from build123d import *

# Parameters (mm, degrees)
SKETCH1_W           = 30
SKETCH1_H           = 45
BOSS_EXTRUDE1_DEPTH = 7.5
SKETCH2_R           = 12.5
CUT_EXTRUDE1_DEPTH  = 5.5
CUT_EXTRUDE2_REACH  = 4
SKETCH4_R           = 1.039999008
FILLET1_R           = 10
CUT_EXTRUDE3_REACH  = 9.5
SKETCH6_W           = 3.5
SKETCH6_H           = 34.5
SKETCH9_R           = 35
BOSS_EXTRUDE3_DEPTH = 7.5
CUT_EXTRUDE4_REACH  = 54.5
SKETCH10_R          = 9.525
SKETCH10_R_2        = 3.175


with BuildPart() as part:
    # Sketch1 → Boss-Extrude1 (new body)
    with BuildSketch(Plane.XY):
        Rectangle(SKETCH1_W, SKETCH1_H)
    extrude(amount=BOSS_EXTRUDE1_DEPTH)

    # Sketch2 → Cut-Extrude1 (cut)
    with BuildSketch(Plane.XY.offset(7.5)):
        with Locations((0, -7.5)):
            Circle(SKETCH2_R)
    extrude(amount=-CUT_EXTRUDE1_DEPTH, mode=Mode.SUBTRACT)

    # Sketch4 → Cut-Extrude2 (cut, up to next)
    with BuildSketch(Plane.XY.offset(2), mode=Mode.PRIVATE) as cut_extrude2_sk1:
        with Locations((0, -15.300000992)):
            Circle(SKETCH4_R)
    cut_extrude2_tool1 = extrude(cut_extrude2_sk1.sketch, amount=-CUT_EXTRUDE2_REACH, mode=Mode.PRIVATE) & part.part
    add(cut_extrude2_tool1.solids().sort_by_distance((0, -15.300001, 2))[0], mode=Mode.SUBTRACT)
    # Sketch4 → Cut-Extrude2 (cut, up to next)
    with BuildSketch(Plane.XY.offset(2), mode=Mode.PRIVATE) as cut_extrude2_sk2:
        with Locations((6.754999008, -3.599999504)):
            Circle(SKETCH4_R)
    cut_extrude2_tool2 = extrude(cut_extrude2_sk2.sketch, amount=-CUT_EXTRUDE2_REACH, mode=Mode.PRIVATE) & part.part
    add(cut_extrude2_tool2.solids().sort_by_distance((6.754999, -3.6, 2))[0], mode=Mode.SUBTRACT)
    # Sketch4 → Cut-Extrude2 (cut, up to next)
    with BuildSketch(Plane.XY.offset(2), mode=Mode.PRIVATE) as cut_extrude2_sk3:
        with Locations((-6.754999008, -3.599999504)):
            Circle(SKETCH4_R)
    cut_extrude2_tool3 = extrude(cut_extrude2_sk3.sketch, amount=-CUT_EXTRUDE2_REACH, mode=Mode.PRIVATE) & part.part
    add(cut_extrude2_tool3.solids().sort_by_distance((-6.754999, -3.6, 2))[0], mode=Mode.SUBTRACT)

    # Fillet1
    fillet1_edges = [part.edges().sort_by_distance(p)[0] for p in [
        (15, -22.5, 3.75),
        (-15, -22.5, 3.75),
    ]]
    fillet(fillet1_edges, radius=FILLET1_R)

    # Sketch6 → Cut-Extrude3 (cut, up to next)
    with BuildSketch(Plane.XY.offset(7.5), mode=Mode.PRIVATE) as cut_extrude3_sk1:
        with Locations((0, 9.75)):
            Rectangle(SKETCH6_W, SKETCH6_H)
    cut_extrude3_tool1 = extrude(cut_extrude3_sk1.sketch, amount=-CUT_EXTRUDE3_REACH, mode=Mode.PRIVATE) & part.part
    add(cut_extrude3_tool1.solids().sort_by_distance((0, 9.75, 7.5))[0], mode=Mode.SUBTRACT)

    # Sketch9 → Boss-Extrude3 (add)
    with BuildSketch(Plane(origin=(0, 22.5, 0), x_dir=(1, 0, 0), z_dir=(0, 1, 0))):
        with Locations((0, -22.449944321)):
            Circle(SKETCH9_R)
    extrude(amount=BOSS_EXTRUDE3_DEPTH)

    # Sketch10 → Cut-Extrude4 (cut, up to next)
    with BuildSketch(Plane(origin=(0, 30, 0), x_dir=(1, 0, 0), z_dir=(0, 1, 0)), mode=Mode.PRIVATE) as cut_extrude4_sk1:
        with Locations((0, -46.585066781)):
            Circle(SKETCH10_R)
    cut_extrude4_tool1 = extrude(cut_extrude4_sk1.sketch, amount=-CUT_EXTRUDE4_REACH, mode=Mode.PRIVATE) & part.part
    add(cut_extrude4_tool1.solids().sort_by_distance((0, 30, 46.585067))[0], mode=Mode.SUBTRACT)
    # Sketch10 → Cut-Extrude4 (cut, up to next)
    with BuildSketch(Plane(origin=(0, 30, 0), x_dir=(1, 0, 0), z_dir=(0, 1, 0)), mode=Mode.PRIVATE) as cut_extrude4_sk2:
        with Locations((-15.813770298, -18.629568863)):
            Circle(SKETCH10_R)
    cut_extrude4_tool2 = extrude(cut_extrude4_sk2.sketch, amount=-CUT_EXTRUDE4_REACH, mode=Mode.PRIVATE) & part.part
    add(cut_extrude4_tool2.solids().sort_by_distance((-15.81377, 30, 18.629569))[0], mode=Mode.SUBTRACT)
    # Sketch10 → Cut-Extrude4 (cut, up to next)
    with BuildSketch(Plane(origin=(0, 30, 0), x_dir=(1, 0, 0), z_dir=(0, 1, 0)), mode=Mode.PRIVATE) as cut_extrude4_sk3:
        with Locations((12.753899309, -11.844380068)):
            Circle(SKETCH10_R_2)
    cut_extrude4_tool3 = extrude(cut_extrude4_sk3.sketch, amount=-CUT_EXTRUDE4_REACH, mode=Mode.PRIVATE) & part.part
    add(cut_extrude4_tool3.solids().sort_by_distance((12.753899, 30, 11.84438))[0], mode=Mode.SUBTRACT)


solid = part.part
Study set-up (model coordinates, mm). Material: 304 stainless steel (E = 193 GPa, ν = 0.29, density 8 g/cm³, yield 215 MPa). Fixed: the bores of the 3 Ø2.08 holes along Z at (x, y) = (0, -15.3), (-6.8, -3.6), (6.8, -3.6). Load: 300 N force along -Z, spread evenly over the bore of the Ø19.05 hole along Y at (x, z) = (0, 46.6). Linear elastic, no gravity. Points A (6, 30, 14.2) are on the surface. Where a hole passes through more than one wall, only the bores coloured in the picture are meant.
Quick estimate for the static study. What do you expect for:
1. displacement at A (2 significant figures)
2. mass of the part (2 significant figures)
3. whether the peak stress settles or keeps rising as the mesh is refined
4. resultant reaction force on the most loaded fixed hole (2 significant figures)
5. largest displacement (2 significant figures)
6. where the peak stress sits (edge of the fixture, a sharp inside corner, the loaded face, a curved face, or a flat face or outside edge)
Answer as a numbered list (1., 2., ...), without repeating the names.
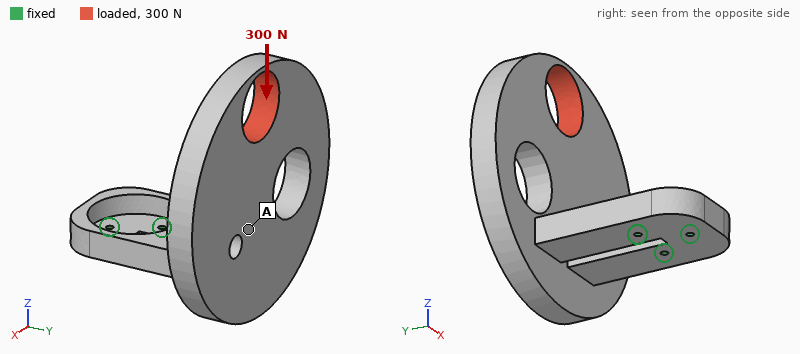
1. 0.096 mm
2. 250 g
3. keeps rising
4. 480 N
5. 0.18 mm
6. edge of the fixture
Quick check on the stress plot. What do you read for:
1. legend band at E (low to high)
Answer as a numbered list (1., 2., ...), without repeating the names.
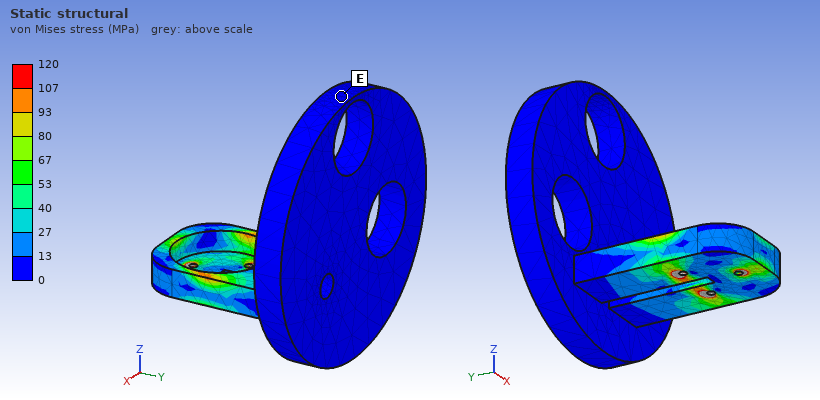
1. 0 to 13 MPa
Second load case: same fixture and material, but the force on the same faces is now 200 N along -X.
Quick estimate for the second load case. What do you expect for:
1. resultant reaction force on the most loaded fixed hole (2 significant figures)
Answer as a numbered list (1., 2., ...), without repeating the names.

1. 570 N
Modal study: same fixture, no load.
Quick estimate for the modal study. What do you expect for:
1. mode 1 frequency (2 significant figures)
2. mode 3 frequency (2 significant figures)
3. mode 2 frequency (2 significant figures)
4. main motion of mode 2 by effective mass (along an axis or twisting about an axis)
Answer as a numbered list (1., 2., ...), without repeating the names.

1. 490 Hz
2. 2100 Hz
3. 640 Hz
4. along X
